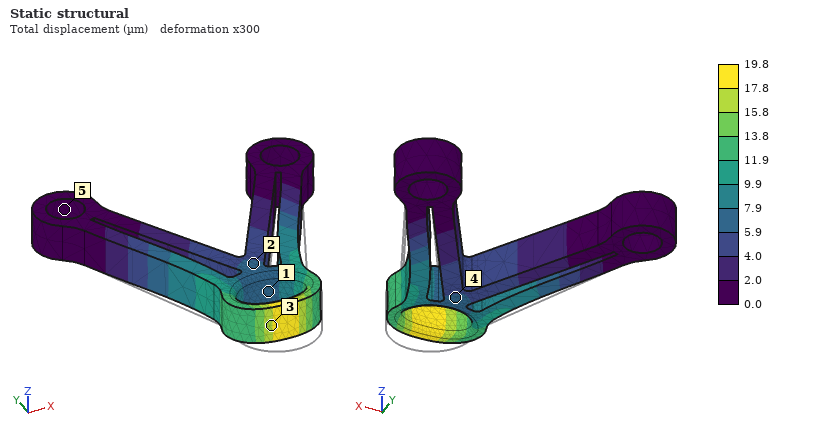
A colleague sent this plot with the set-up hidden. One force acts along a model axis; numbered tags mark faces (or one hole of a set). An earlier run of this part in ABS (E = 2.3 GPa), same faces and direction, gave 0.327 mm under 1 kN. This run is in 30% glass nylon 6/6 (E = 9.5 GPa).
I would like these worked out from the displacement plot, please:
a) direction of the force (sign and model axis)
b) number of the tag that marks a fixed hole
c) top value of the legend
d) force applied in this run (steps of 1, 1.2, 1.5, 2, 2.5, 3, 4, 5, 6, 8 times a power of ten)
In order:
+Y
5
19.8 µm
250 N
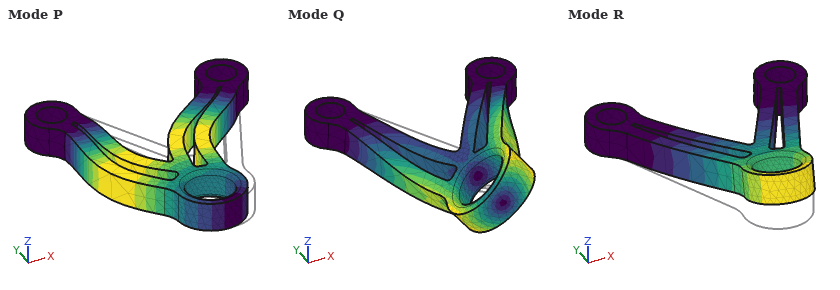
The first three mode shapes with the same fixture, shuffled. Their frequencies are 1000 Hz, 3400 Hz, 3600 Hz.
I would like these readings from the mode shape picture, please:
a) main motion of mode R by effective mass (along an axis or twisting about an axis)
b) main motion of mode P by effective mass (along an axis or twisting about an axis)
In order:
along Z
along X
